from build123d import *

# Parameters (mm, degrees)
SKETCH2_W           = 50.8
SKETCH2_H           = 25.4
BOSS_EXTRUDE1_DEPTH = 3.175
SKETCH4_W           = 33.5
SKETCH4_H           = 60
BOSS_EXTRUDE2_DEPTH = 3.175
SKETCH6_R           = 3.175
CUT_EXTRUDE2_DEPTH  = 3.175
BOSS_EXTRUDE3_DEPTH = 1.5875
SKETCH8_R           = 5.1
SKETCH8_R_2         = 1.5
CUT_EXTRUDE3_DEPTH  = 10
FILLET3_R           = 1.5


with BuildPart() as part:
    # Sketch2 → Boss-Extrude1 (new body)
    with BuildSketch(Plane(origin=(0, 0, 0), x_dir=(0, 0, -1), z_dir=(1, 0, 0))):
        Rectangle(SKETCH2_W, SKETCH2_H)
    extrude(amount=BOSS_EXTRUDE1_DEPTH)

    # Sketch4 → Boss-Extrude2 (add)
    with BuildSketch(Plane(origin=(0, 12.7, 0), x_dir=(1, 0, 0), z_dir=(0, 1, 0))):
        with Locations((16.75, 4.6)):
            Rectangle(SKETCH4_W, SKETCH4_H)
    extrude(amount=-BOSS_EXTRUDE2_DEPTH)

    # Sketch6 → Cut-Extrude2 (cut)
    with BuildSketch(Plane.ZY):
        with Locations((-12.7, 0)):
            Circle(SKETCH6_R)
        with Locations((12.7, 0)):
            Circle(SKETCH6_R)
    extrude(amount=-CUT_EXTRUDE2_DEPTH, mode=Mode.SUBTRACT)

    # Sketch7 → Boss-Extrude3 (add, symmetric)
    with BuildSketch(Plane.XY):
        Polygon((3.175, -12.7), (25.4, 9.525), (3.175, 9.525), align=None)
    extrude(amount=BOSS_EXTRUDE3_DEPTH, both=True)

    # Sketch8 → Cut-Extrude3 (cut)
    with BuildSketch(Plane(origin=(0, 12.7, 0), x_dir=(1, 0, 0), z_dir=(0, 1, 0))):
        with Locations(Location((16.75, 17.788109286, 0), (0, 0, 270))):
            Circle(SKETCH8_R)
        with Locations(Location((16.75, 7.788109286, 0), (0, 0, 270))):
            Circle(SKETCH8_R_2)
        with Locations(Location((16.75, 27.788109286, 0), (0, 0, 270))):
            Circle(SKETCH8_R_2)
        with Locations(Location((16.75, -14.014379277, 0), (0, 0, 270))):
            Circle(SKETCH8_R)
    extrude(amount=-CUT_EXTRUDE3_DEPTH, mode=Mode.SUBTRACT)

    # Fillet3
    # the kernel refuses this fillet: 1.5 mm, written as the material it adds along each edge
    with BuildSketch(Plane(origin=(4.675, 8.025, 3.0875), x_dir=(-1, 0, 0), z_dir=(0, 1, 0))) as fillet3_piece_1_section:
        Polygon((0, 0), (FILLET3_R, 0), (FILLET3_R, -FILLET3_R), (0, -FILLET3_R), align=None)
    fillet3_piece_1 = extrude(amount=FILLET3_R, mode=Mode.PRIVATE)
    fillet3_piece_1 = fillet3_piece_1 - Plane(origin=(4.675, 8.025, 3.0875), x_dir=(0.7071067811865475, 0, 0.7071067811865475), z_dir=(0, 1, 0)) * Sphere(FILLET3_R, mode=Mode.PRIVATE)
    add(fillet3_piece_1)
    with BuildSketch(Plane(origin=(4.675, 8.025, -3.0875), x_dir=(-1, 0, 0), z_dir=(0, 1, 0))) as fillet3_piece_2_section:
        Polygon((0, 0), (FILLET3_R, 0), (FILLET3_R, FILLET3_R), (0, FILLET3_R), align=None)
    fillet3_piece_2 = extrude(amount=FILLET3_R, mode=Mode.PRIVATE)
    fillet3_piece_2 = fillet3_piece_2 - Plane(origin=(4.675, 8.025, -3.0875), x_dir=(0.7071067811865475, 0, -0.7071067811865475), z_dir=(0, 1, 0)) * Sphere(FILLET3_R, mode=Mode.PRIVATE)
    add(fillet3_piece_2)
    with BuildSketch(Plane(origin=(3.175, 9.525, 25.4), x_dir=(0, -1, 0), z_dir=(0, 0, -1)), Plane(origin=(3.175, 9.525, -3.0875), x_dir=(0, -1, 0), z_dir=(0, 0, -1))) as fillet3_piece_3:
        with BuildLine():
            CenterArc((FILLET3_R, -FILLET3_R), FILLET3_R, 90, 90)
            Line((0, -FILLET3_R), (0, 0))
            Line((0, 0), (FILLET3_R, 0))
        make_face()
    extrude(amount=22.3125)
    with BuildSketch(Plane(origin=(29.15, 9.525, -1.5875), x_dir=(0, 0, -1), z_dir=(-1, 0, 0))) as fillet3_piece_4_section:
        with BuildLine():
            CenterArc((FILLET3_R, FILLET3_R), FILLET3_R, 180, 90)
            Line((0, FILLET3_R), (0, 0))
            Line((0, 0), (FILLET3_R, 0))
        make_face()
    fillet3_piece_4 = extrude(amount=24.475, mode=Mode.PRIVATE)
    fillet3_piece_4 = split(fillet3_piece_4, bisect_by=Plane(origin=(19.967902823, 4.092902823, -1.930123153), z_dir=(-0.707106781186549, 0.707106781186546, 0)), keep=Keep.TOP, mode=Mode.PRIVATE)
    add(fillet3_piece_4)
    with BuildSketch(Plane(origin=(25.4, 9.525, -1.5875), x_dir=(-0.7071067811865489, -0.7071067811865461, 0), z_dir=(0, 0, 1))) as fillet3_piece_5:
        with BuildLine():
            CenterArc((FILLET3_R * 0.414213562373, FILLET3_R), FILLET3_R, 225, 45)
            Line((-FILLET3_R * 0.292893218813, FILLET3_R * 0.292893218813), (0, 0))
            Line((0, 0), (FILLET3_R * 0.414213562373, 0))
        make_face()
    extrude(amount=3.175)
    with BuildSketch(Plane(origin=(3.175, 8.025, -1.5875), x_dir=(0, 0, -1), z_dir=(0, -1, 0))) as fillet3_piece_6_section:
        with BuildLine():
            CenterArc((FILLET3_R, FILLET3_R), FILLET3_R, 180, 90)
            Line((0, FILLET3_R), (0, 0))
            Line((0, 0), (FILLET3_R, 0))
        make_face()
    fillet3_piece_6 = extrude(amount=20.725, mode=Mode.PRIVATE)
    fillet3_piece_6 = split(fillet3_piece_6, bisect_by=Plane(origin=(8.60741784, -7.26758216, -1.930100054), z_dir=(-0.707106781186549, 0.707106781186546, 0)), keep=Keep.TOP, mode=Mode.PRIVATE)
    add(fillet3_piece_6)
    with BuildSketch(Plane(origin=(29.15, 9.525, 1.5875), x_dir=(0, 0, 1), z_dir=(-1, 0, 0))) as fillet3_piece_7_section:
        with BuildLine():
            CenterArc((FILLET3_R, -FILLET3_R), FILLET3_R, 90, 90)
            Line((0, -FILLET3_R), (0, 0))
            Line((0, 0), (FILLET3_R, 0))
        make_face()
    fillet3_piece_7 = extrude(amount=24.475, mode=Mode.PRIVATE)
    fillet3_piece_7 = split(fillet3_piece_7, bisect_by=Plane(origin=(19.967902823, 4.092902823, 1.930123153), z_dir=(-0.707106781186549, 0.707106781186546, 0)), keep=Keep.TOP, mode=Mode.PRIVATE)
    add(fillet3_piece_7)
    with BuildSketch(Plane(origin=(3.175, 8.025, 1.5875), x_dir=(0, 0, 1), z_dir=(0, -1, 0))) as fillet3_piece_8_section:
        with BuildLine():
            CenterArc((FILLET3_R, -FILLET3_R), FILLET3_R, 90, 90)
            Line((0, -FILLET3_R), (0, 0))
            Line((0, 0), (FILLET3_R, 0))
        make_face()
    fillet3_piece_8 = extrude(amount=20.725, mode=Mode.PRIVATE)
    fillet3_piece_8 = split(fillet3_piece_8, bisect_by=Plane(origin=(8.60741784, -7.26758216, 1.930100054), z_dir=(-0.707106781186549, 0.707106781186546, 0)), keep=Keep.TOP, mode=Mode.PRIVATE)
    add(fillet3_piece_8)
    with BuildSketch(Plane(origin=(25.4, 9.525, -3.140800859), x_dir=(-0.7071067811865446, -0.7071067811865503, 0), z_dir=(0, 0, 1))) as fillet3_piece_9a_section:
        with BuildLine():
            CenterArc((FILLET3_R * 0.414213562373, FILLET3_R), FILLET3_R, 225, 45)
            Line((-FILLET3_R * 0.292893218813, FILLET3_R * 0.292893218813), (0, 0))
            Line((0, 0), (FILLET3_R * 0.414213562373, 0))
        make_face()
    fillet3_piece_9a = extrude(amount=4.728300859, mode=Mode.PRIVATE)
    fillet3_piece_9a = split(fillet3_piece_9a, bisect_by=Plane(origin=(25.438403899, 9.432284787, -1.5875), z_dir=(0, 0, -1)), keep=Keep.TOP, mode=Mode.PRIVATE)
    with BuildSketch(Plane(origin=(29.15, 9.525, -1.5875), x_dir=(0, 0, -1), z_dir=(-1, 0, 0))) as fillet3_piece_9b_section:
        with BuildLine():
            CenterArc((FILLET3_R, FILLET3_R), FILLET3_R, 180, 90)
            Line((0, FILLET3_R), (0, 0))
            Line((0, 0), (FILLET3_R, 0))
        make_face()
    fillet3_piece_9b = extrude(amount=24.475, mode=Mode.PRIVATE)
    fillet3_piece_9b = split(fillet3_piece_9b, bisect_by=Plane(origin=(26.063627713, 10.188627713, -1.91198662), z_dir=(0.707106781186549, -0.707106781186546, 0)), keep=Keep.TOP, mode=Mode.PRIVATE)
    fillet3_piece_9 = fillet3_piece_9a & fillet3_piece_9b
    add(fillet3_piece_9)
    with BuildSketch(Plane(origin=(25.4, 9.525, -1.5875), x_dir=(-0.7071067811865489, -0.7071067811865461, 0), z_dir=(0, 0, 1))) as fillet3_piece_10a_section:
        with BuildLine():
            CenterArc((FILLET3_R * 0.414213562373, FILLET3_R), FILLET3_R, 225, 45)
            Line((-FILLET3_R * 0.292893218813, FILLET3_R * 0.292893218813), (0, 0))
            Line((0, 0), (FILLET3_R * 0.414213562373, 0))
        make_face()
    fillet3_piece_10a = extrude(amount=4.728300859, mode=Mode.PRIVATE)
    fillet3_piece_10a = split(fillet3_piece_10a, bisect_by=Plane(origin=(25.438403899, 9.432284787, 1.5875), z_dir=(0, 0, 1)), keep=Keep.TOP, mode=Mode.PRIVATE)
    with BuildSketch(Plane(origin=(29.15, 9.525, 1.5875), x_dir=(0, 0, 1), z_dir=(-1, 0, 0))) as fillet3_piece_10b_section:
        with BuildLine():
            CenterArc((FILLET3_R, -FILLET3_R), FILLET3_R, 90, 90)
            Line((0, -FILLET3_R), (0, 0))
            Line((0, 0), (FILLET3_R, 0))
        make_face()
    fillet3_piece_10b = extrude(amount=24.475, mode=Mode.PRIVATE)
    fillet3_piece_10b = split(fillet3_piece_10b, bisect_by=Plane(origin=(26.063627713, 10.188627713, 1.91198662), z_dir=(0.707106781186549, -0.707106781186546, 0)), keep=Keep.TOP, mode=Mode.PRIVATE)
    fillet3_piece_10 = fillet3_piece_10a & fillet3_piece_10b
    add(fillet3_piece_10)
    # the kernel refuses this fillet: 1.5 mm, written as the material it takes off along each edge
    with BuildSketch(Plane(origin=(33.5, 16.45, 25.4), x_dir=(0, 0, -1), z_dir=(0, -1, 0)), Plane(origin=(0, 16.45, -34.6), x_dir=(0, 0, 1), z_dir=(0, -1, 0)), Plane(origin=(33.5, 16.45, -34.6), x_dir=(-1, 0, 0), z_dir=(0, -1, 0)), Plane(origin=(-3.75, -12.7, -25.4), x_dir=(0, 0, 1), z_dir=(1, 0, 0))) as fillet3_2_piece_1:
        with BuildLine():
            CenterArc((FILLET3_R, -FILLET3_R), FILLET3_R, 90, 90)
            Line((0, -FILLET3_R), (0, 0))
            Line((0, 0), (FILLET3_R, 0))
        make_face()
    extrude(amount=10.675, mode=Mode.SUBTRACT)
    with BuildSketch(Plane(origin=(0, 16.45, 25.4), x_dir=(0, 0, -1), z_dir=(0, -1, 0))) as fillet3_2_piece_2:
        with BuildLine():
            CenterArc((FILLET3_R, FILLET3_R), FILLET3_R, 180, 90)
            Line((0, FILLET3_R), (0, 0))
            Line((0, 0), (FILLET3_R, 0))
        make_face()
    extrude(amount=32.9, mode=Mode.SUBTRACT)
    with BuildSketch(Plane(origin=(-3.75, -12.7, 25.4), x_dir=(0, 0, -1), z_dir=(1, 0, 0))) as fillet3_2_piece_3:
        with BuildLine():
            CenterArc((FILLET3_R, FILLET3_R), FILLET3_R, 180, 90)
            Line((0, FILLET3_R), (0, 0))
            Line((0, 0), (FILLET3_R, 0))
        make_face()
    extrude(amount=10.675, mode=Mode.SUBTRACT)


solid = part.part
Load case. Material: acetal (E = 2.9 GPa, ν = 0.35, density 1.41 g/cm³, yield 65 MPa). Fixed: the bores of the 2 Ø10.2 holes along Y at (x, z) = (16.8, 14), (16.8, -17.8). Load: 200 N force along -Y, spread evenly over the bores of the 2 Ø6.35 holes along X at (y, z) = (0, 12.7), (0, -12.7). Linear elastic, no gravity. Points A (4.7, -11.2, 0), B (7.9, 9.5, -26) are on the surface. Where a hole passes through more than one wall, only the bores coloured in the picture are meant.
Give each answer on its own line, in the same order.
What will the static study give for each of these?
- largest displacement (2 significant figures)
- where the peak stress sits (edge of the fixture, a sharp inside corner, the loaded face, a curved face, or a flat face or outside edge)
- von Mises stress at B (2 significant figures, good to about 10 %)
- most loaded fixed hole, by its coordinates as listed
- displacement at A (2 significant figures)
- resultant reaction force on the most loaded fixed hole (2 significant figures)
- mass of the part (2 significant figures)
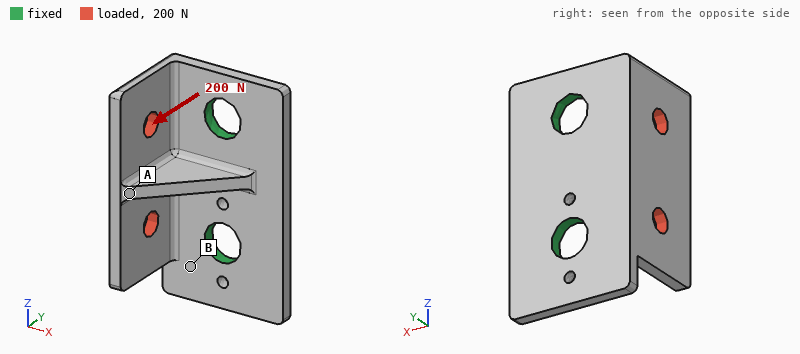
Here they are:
0.45 mm
a flat face or outside edge
6.3 MPa
(16.8, 14)
0.32 mm
120 N
14 g
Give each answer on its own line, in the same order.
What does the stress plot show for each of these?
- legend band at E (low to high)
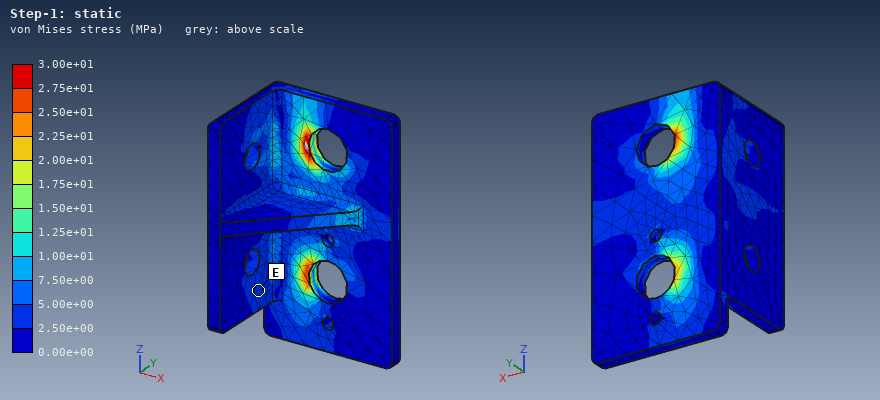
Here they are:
2.50e+00 to 5.00e+00 MPa
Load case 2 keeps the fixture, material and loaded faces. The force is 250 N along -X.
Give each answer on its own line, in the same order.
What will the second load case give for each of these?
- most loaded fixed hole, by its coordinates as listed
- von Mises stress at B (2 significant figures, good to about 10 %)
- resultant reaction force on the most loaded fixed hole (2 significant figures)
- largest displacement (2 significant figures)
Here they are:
(16.8, 14)
9.0 MPa
140 N
0.80 mm
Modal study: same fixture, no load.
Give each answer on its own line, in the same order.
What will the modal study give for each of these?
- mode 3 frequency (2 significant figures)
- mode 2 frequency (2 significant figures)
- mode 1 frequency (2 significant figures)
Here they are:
2400 Hz
1600 Hz
1300 Hz
